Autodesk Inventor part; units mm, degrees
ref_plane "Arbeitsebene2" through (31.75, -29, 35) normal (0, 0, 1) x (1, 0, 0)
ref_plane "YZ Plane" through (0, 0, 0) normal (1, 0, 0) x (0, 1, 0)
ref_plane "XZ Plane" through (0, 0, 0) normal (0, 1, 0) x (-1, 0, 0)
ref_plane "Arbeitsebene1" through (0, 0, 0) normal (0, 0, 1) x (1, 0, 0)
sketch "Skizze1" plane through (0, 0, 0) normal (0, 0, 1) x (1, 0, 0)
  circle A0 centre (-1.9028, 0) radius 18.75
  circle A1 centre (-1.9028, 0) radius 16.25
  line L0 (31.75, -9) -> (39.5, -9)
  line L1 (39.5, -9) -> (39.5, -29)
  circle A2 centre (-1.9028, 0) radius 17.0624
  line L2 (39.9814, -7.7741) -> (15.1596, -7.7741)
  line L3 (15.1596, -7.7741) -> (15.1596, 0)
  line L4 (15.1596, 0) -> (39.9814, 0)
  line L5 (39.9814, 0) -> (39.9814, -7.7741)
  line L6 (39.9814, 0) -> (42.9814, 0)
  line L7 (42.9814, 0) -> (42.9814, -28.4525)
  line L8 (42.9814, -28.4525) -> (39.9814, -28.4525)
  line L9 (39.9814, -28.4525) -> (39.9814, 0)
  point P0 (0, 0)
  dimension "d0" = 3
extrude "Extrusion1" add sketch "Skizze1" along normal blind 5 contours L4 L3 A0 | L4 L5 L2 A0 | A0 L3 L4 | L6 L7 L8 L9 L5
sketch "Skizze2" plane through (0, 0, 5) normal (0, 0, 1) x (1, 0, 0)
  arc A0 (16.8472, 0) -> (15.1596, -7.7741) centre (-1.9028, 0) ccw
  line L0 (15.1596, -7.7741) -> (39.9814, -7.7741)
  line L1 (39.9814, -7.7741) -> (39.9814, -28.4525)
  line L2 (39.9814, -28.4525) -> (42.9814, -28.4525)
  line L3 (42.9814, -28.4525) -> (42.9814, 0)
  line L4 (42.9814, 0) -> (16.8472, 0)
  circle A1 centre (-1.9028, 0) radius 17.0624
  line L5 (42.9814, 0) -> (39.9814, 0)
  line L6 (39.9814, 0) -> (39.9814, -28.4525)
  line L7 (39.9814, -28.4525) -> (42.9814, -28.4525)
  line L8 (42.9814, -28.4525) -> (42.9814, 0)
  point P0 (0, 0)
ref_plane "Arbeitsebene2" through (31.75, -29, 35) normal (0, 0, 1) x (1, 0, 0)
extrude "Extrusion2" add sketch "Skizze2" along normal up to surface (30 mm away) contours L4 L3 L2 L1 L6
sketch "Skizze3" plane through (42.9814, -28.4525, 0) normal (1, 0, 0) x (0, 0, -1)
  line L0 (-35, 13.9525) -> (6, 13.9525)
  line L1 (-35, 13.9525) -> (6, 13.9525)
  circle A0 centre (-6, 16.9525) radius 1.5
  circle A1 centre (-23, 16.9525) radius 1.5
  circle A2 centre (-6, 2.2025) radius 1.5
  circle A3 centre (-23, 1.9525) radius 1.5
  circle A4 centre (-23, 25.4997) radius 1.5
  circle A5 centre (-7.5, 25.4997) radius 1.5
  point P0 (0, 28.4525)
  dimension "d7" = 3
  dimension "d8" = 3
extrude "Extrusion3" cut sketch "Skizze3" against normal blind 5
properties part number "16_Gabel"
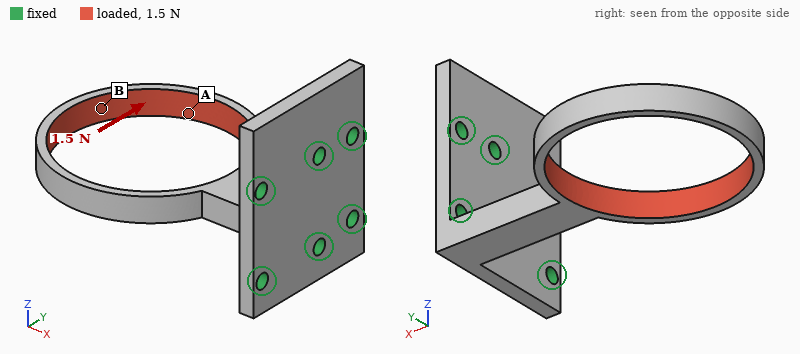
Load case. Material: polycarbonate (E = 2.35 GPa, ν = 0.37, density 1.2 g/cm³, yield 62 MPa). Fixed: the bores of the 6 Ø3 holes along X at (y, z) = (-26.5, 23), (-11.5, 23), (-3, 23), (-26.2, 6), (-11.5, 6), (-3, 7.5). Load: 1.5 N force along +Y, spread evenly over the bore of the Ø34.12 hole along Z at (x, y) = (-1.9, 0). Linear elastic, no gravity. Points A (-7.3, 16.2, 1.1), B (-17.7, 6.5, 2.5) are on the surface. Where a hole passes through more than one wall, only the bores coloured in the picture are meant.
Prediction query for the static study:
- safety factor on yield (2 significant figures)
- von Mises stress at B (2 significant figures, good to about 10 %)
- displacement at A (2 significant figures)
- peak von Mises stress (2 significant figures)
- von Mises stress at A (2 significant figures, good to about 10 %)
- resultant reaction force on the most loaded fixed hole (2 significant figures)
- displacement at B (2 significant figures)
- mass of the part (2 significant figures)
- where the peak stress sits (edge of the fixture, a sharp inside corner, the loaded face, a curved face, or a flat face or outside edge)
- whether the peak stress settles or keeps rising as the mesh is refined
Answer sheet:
12
0.65 MPa
0.76 mm
5.0 MPa
1.7 MPa
6.8 N
0.90 mm
5.7 g
the loaded face
settles
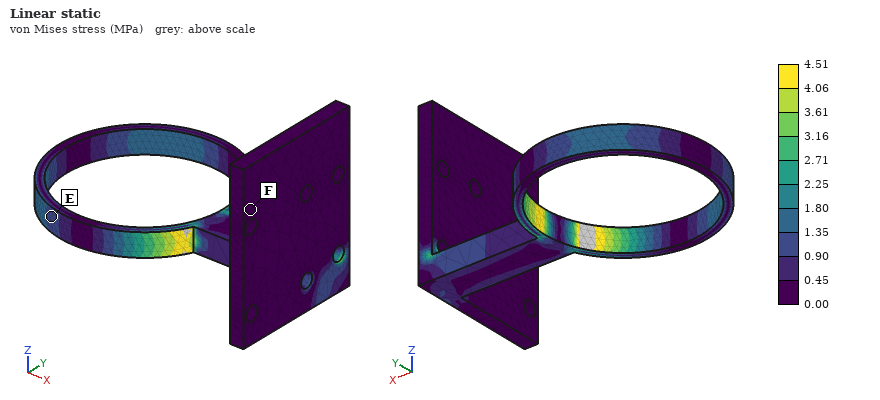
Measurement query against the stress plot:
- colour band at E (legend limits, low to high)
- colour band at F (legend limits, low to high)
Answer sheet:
0.90 to 1.35 MPa
0.00 to 0.45 MPa
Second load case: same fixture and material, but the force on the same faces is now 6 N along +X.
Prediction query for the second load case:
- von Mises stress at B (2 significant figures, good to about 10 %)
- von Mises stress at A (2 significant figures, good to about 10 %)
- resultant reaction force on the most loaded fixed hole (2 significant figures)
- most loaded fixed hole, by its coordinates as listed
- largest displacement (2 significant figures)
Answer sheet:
2.6 MPa
2.7 MPa
6.9 N
(-3, 7.5)
0.82 mm
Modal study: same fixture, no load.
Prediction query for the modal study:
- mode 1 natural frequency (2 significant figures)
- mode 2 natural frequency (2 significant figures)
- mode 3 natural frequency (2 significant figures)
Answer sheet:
200 Hz
210 Hz
620 Hz
